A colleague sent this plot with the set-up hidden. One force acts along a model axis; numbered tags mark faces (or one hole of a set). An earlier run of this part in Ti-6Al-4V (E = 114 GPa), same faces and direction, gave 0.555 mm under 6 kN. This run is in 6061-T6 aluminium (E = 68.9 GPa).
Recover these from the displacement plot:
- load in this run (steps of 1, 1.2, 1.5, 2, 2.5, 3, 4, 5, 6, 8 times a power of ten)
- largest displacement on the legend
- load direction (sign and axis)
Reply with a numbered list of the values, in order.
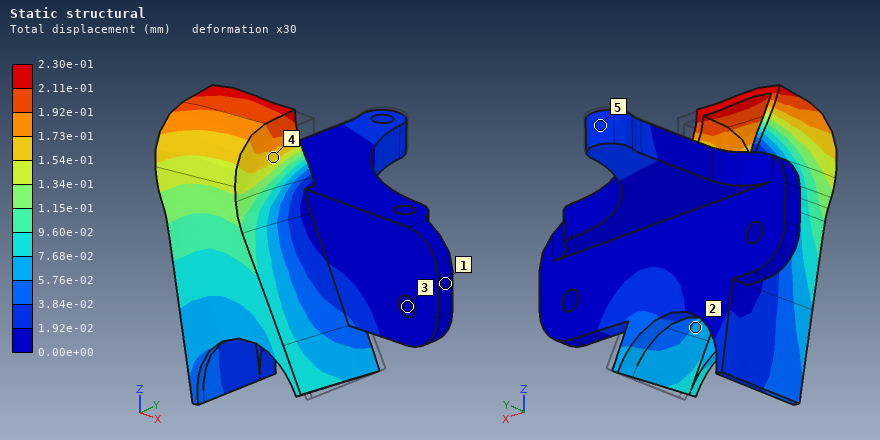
1. 1.5 kN
2. 2.30e-01 mm
3. -X
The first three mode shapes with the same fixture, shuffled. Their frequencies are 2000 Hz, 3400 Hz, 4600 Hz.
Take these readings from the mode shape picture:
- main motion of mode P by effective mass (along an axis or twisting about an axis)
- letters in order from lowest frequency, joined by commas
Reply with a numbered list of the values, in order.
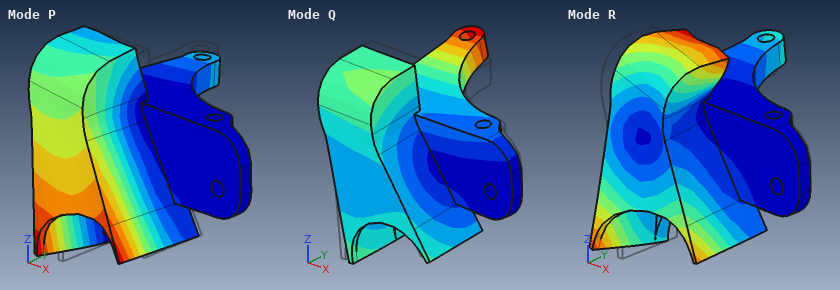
1. along X
2. Q, P, R
